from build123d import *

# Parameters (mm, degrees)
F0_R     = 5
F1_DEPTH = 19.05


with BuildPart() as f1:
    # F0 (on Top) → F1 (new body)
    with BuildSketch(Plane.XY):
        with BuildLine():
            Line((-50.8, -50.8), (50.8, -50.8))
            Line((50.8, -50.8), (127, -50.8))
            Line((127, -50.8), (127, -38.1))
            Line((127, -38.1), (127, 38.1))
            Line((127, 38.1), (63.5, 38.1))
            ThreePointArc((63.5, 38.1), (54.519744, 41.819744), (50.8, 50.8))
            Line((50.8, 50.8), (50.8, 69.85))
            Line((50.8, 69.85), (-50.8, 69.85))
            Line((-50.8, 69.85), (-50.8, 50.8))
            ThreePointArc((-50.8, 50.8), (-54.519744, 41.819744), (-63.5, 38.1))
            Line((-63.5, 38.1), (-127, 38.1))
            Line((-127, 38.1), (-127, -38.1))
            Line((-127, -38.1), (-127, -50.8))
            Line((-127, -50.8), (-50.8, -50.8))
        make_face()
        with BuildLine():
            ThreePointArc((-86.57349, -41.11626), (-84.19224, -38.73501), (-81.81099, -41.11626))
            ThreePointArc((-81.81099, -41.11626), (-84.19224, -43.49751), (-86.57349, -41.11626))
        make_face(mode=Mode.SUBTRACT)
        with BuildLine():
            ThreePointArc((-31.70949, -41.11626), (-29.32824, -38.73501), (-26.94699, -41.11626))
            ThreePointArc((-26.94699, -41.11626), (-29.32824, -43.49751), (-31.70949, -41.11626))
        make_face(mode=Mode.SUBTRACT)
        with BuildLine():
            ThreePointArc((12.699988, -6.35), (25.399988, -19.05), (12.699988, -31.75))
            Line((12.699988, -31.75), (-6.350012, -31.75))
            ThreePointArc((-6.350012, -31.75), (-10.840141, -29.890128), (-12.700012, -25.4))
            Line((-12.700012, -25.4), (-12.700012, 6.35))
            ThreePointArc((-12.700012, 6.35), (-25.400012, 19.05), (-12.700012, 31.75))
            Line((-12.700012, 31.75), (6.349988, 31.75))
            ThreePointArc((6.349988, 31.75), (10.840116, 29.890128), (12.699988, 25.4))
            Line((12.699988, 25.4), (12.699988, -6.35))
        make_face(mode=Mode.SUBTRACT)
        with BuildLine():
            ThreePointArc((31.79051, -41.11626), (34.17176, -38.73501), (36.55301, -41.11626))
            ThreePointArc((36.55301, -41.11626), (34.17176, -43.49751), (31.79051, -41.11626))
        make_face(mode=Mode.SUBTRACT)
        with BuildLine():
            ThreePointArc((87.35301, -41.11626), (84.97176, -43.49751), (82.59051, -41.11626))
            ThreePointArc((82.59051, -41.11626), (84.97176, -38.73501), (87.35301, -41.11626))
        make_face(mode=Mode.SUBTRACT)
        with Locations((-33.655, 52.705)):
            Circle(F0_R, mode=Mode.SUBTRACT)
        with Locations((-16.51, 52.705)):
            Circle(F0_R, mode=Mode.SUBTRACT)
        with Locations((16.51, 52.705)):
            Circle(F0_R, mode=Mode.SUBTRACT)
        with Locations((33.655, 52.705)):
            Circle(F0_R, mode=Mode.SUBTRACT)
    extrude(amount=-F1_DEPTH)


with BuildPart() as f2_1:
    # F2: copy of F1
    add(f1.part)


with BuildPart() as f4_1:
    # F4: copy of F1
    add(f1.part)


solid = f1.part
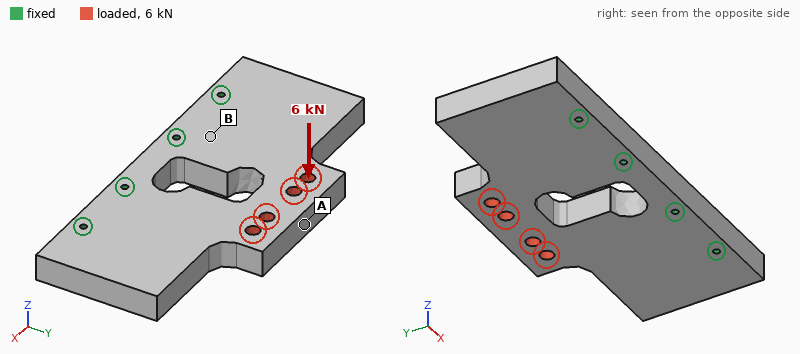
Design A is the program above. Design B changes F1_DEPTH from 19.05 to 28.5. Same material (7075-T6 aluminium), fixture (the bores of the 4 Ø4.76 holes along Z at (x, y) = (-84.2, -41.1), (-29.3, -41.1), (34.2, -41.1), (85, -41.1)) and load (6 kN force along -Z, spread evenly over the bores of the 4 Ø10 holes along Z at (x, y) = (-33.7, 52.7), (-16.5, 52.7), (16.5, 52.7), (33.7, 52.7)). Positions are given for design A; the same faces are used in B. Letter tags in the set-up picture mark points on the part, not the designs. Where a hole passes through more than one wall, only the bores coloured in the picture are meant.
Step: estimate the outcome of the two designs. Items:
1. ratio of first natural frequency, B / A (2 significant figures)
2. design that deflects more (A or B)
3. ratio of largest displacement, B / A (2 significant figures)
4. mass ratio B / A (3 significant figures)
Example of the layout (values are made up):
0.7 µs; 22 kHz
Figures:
1.4; A; 0.33; 1.50
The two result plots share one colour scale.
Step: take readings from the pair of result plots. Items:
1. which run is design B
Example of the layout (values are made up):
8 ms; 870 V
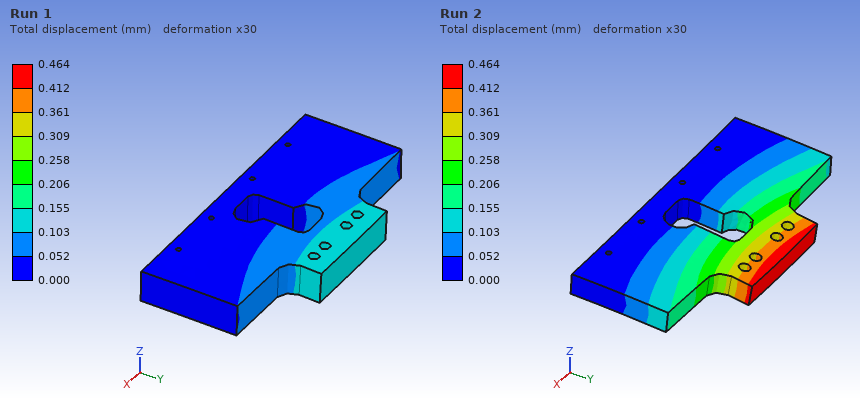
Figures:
Run 1
